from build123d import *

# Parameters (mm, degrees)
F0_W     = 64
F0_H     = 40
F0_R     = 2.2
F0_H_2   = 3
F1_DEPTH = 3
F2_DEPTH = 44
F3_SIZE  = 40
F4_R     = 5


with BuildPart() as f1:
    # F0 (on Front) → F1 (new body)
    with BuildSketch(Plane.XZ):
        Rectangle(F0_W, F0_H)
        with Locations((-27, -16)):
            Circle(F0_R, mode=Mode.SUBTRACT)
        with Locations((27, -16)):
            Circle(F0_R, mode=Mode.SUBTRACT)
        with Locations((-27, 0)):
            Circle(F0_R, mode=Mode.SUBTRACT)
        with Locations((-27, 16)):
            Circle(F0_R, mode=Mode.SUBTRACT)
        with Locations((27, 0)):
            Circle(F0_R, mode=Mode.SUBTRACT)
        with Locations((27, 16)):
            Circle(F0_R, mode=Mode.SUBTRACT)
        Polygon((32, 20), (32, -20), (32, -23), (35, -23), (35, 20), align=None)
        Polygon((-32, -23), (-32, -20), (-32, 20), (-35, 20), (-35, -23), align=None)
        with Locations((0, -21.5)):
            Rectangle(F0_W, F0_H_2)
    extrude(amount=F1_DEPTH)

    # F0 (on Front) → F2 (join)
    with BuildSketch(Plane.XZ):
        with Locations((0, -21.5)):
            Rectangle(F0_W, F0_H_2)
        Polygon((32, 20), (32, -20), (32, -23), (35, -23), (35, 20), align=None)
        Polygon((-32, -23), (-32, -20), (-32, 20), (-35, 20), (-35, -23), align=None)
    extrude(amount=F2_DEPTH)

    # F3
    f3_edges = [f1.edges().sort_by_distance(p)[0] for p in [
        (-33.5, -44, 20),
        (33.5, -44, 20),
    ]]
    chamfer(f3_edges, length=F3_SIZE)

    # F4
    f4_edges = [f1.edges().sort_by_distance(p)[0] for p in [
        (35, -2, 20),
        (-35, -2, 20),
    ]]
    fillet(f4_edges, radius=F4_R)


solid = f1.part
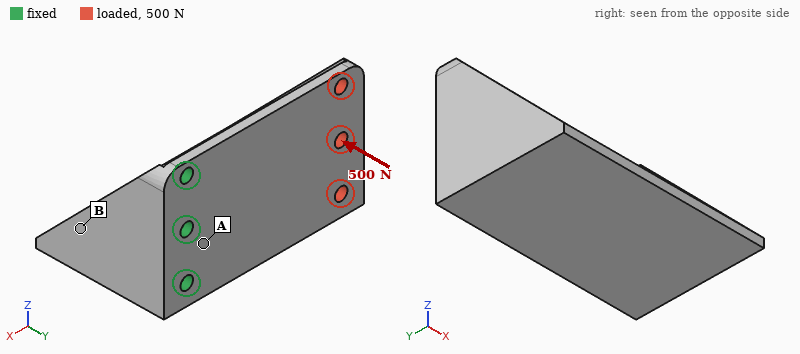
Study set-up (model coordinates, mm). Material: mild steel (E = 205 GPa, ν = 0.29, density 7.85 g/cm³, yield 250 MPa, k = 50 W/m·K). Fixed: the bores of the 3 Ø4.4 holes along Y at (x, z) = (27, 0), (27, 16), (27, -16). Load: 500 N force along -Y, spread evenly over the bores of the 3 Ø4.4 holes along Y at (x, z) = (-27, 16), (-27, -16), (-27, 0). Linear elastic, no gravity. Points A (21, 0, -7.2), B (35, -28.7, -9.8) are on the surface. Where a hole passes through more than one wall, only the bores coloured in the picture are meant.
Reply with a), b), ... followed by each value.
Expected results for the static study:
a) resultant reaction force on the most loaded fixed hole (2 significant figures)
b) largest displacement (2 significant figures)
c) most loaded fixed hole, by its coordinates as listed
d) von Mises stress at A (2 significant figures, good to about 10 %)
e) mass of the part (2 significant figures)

a) 400 N
b) 0.40 mm
c) (27, 16)
d) 110 MPa
e) 180 g
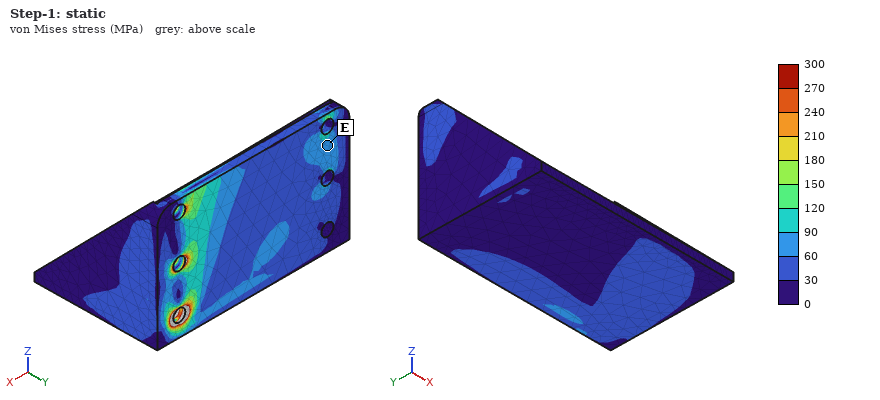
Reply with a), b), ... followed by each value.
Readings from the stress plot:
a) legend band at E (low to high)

a) 60 to 90 MPa
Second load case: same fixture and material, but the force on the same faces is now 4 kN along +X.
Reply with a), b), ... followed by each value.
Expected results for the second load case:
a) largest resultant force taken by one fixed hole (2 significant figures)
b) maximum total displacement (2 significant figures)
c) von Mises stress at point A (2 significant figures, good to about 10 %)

a) 1.4 kN
b) 13 µm
c) 19 MPa
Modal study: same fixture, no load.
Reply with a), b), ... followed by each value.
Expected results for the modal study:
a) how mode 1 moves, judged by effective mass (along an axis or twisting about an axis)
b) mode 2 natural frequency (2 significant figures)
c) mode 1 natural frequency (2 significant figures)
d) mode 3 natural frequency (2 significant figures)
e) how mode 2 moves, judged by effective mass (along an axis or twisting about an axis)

a) along Y
b) 1100 Hz
c) 770 Hz
d) 3300 Hz
e) along Z
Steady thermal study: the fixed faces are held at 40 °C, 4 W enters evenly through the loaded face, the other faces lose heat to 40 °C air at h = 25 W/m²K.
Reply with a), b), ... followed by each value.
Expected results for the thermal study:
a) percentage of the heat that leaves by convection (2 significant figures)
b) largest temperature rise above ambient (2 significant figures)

a) 55 %
b) 17 K
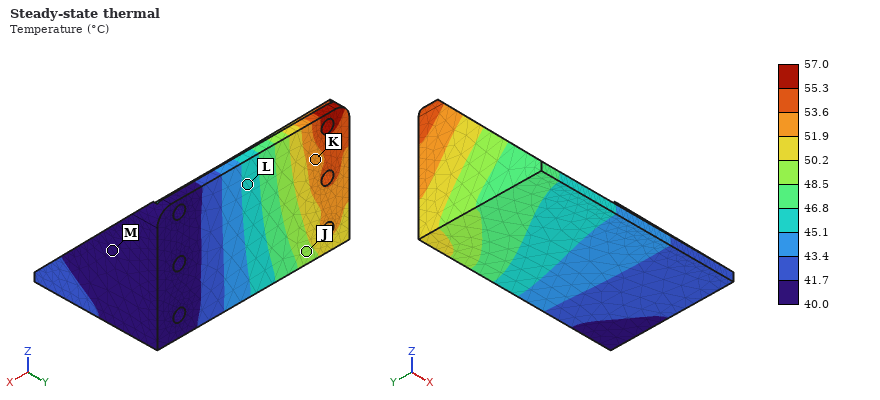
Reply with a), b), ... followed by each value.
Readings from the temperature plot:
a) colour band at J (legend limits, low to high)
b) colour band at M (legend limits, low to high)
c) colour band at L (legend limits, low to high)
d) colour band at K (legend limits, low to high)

a) 48.5 to 50.2 °C
b) 40.0 to 41.7 °C
c) 45.1 to 46.8 °C
d) 51.9 to 53.6 °C
